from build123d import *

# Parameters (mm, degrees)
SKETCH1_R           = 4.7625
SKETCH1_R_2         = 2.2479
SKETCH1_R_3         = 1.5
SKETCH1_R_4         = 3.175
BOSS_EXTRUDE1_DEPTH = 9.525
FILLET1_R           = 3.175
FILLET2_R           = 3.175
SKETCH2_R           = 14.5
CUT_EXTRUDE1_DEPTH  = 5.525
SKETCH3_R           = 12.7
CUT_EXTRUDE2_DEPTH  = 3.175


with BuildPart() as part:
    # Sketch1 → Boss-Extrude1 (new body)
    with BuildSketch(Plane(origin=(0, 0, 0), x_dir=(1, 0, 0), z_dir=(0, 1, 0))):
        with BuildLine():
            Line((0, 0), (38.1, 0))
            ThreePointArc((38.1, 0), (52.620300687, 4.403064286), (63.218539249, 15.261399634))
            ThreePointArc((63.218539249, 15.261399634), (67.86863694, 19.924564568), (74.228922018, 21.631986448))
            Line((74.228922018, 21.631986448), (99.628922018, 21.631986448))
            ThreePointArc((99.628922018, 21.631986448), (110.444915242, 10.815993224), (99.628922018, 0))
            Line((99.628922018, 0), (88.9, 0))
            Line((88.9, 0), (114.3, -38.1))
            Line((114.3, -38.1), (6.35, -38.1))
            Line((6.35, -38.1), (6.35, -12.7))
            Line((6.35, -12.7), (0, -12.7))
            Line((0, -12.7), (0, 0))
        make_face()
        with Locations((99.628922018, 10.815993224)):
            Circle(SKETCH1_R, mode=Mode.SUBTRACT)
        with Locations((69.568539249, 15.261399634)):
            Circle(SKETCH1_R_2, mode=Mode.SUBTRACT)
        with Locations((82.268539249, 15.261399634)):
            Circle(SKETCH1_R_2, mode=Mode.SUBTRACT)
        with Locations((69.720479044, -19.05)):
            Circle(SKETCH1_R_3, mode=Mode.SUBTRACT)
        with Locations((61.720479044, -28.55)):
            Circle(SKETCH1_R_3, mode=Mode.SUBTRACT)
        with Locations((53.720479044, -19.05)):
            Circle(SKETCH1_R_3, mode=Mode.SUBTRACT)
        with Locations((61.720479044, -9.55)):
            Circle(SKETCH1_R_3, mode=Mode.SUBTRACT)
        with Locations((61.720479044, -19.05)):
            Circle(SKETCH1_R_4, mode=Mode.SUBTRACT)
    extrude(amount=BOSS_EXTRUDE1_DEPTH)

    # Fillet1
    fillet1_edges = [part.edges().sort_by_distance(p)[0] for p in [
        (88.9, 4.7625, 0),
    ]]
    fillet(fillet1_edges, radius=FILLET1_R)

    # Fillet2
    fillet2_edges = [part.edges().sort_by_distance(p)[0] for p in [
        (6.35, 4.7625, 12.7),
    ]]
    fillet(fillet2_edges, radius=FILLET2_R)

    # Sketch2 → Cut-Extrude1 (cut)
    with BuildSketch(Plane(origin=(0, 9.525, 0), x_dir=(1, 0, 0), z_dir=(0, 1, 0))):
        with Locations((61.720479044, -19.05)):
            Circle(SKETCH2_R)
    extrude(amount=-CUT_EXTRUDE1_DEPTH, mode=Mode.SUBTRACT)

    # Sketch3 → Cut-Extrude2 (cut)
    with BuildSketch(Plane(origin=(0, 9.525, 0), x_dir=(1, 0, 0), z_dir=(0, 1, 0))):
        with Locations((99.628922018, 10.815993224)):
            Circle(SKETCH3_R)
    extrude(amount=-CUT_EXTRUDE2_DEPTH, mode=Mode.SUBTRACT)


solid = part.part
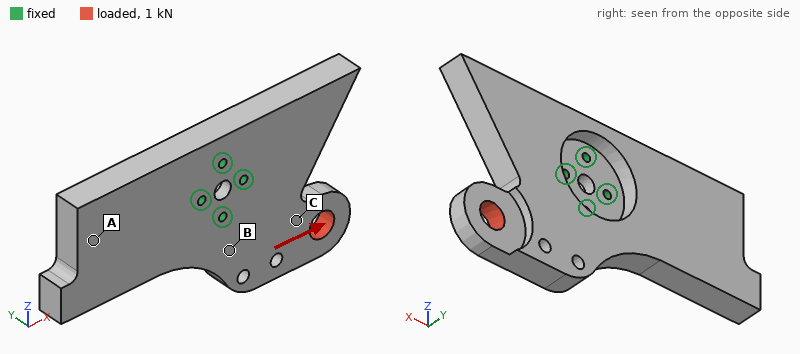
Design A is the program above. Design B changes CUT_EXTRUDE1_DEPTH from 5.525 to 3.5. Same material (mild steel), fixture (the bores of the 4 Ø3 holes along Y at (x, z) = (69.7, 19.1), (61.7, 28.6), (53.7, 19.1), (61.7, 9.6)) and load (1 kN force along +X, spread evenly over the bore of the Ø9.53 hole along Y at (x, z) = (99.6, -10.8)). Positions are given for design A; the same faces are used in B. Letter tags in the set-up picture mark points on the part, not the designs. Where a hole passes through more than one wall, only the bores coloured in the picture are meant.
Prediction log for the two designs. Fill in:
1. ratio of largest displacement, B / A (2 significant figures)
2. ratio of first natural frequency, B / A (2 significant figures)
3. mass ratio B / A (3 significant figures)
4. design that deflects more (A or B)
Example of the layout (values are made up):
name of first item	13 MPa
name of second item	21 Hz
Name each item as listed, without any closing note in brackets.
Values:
ratio of largest displacement, B / A	0.87
ratio of first natural frequency, B / A	1.3
mass ratio B / A	1.03
design that deflects more	A
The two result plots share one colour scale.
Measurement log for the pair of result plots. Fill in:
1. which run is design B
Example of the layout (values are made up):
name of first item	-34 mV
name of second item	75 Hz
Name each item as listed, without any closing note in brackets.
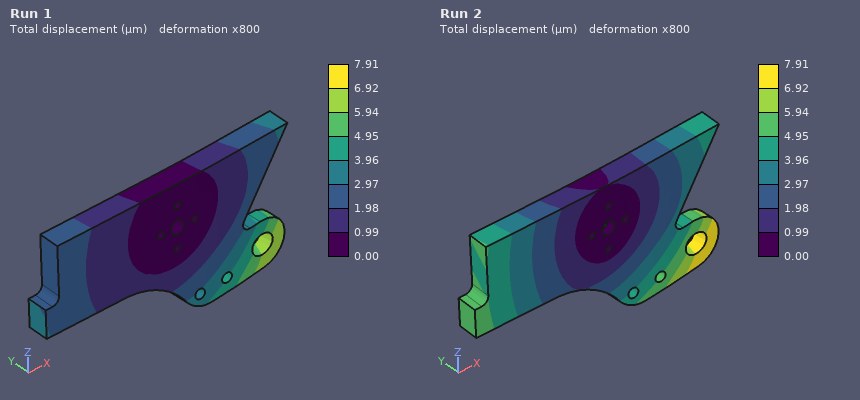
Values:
which run is design B	Run 1
